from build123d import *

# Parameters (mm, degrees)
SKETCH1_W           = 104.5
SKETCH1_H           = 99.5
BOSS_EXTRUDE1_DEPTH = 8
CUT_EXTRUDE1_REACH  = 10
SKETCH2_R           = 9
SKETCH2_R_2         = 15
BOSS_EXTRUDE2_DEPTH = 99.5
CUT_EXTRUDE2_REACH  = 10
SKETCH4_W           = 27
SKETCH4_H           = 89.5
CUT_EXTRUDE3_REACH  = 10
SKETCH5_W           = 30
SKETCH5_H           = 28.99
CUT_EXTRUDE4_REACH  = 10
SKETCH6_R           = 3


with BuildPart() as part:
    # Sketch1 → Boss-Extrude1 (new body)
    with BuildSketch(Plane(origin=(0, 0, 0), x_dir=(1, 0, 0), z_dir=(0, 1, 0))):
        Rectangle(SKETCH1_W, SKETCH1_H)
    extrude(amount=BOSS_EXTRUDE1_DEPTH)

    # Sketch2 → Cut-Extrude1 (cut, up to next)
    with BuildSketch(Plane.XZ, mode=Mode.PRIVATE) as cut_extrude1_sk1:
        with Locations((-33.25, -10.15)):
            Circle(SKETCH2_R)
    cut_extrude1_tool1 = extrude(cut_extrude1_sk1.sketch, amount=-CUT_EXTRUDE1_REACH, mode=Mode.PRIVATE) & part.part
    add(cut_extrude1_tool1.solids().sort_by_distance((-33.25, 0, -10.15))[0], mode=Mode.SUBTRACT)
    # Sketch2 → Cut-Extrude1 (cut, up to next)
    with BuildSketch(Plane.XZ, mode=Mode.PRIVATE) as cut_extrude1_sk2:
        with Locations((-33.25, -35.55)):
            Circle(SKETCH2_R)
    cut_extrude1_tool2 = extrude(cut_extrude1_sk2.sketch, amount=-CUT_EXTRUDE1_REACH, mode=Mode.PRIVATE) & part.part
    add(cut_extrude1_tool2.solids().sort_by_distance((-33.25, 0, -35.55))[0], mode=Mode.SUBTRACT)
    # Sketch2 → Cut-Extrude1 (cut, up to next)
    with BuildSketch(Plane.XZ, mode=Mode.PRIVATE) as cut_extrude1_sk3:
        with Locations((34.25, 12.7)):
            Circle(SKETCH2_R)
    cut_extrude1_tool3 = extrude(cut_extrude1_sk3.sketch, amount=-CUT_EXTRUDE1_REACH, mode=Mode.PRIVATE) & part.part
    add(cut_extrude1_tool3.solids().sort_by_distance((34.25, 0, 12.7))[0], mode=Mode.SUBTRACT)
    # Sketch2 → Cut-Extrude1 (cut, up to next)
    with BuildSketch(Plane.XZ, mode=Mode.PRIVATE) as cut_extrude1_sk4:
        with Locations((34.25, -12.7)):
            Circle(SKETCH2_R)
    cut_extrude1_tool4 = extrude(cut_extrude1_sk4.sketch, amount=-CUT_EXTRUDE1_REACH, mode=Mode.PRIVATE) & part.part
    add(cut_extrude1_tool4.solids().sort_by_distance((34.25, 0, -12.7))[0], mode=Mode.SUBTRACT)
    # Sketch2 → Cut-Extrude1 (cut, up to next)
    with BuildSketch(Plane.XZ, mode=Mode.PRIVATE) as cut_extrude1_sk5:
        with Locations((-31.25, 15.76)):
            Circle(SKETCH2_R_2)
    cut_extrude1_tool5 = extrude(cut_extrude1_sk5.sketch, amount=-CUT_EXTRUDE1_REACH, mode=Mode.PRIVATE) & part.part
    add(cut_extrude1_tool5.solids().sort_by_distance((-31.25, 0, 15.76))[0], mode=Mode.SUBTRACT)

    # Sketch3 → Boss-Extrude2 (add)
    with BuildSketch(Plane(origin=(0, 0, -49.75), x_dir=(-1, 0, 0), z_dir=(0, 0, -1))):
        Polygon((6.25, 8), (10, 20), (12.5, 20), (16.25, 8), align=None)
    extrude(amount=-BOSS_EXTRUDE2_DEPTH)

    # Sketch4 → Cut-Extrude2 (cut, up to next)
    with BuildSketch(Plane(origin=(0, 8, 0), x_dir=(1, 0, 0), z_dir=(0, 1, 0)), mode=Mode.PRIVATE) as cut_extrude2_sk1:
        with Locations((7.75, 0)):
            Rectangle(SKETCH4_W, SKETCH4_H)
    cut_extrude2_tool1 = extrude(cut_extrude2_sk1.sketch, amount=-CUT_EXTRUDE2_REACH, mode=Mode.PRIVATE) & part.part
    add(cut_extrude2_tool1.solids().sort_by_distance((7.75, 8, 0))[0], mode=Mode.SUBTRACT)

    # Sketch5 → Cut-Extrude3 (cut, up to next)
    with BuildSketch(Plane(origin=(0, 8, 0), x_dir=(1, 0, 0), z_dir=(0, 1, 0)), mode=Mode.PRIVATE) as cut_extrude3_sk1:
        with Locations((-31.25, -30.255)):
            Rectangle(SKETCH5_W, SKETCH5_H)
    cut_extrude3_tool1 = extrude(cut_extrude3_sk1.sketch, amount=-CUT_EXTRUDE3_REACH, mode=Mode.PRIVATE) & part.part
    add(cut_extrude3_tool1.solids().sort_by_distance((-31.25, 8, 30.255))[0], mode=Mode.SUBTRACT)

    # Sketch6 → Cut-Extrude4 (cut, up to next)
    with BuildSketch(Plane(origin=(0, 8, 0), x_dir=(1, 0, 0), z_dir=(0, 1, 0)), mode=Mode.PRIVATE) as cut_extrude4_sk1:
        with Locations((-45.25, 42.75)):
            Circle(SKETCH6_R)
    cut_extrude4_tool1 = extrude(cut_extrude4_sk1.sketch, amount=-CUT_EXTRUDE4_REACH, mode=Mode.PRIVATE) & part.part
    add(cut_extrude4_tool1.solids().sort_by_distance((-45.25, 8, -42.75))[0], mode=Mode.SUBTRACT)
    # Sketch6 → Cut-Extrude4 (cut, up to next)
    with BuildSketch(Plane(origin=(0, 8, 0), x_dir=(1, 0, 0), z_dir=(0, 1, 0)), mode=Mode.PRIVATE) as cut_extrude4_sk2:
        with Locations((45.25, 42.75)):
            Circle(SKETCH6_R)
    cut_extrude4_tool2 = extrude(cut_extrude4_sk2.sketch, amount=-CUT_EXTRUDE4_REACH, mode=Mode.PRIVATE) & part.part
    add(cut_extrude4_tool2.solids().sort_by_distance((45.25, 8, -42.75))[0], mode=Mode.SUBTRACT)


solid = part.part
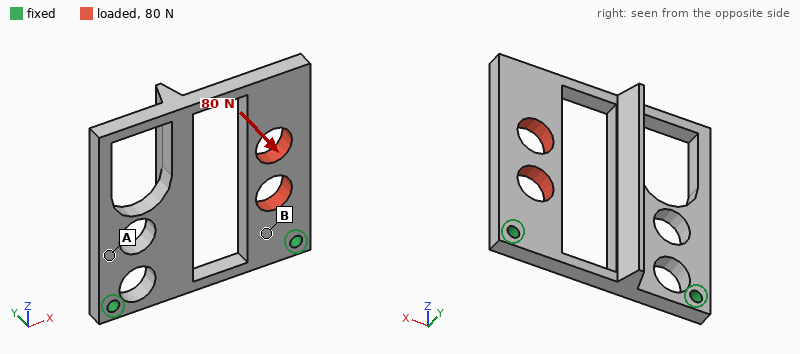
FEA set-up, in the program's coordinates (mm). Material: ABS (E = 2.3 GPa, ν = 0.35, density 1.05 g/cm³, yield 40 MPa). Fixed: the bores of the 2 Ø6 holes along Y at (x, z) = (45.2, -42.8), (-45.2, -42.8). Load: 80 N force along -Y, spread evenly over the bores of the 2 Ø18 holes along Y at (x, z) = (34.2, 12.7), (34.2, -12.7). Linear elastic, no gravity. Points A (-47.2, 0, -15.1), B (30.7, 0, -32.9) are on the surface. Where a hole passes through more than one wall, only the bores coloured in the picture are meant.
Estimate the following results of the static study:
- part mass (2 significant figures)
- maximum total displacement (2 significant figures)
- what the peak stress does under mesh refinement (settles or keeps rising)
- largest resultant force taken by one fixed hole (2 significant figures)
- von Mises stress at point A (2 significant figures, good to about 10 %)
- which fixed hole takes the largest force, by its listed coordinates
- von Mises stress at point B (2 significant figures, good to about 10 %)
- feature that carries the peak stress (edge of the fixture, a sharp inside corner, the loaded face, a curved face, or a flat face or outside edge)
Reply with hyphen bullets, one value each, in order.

- 56 g
- 1.7 mm
- keeps rising
- 76 N
- 1.7 MPa
- (45.2, -42.8)
- 3.7 MPa
- edge of the fixture
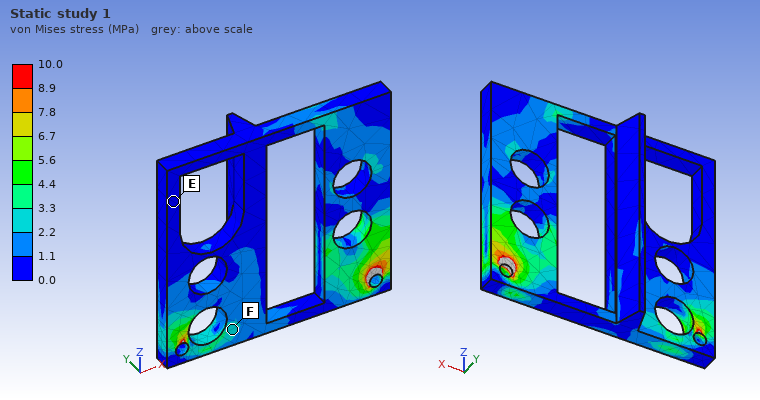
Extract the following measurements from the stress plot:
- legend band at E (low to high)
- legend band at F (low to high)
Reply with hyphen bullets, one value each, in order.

- 0.0 to 1.1 MPa
- 2.2 to 3.3 MPa
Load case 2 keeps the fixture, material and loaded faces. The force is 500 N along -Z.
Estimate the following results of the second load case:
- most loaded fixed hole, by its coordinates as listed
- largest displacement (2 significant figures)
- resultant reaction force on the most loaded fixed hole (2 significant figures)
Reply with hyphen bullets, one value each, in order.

- (45.2, -42.8)
- 0.28 mm
- 470 N
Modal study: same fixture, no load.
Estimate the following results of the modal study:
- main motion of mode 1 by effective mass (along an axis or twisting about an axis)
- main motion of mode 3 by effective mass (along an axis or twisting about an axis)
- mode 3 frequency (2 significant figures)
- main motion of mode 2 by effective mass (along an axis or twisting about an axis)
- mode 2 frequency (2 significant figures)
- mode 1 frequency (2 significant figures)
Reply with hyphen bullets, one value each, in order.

- along Y
- along X
- 490 Hz
- twisting about Z
- 400 Hz
- 170 Hz
